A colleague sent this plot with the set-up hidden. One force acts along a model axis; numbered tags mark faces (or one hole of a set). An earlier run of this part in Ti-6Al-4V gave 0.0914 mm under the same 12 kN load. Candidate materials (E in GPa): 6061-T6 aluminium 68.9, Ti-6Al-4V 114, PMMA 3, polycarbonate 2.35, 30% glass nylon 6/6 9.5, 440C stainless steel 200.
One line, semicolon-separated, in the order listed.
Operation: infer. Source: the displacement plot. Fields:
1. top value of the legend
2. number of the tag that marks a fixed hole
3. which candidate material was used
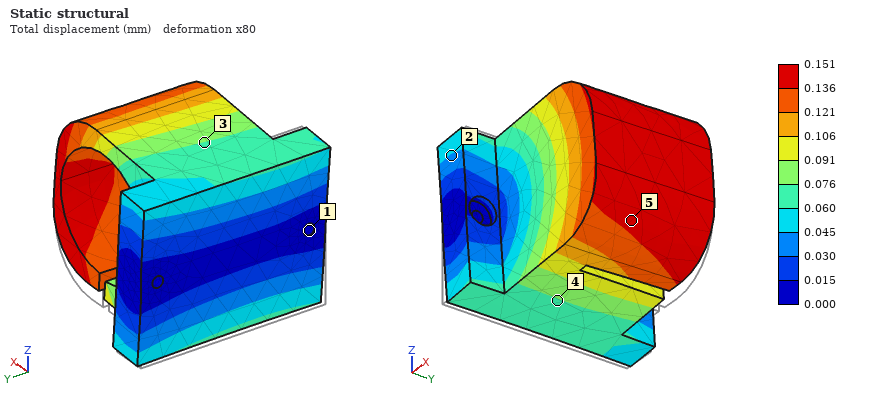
0.151 mm; 1; 6061-T6 aluminium
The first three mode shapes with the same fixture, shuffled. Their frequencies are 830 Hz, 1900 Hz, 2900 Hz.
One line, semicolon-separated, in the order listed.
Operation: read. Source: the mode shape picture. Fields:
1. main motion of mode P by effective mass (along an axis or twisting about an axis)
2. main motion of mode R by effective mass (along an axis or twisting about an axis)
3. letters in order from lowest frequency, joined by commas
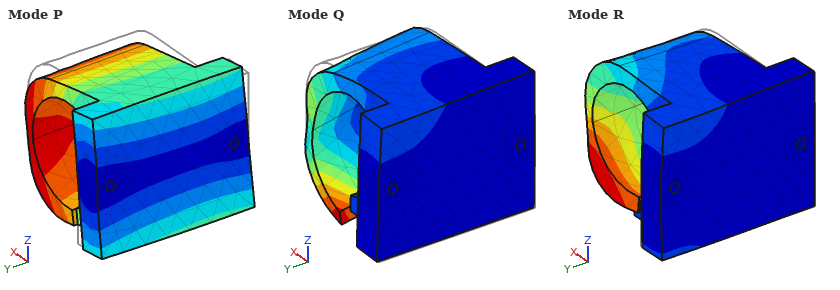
along Z; along Y; P, R, Q
